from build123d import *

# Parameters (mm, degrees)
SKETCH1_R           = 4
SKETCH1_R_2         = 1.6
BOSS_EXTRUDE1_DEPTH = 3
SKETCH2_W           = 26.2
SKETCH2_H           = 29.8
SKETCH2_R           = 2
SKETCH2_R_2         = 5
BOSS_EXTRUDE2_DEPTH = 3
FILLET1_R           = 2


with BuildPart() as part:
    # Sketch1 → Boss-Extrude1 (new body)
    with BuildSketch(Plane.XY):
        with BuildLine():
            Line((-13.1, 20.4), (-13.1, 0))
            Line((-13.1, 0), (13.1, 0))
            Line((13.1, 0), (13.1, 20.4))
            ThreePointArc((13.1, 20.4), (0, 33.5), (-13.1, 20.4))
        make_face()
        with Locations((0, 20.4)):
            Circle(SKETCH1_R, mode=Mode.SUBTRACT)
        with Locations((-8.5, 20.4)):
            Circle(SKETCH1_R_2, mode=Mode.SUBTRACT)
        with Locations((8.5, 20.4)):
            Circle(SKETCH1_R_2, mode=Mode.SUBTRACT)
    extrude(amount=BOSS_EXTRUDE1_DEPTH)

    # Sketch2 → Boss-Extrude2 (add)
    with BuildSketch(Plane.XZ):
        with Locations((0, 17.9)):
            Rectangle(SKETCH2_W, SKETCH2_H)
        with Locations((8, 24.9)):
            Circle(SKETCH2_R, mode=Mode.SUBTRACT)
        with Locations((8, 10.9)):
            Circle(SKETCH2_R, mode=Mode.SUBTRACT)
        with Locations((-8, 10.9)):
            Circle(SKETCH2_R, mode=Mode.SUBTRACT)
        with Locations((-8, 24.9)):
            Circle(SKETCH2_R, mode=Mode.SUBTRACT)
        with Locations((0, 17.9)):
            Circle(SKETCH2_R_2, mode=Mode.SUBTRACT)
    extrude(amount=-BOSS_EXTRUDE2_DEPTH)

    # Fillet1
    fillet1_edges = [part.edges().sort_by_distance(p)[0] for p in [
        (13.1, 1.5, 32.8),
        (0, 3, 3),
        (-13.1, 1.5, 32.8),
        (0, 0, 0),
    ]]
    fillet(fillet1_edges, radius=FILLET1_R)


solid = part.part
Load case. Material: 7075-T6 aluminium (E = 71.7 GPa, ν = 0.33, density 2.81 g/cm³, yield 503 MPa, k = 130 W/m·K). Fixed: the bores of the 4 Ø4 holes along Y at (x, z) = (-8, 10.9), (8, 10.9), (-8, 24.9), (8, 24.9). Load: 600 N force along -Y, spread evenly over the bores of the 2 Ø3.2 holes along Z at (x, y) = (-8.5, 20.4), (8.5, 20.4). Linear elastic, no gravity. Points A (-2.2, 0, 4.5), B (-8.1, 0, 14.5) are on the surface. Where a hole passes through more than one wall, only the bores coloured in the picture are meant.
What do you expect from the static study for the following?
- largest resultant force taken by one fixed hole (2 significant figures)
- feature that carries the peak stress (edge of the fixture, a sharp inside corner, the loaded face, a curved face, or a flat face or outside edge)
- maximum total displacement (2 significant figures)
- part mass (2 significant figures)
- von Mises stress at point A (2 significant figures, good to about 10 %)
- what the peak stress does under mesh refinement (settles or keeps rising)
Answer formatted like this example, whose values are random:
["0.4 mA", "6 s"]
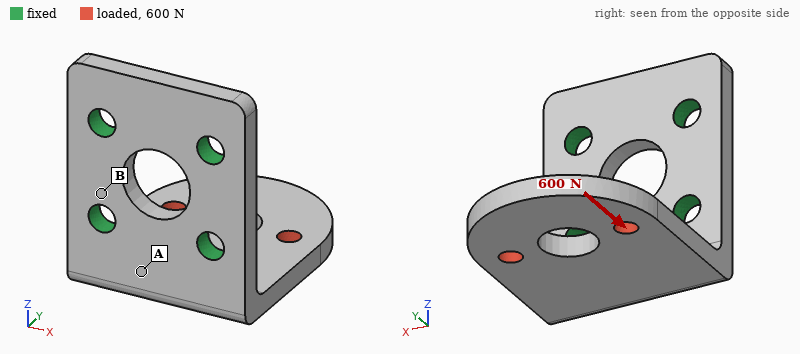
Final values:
["310 N", "edge of the fixture", "0.17 mm", "12 g", "38 MPa", "keeps rising"]
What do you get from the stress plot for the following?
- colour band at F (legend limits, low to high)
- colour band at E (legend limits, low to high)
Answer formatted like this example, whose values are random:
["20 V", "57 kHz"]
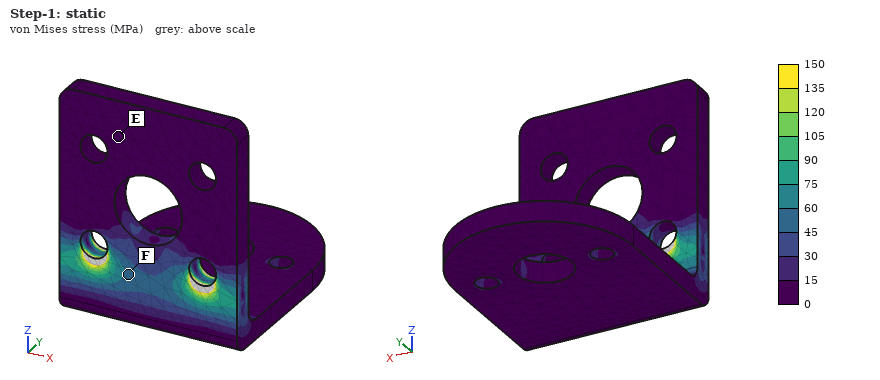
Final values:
["45 to 60 MPa", "0 to 15 MPa"]
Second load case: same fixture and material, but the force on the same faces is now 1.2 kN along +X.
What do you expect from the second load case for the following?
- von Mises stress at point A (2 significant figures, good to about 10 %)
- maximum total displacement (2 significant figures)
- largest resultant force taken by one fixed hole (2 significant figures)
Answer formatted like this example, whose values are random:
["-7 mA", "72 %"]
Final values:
["120 MPa", "0.28 mm", "1.5 kN"]
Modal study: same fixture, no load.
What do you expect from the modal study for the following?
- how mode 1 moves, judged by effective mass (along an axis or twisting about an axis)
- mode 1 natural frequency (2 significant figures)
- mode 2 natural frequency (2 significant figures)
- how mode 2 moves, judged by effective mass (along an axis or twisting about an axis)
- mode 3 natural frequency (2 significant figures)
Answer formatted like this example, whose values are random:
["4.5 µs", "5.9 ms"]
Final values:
["along Z", "2200 Hz", "5500 Hz", "along X", "8300 Hz"]
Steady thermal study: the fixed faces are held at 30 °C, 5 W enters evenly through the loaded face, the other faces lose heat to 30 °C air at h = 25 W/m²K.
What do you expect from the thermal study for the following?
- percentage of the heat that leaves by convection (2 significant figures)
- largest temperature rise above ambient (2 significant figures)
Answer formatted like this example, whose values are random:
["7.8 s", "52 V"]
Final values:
["8.7 %", "14 K"]
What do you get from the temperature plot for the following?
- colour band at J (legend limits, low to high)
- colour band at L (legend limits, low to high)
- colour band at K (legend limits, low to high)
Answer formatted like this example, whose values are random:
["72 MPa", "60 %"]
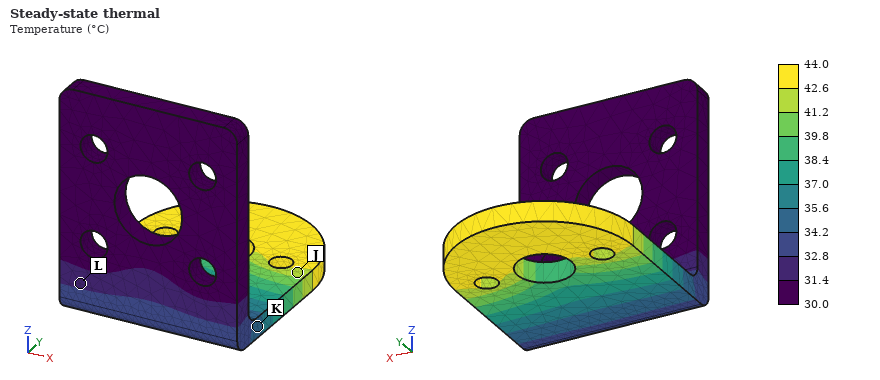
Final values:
["41.2 to 42.6 °C", "31.4 to 32.8 °C", "34.2 to 35.6 °C"]
